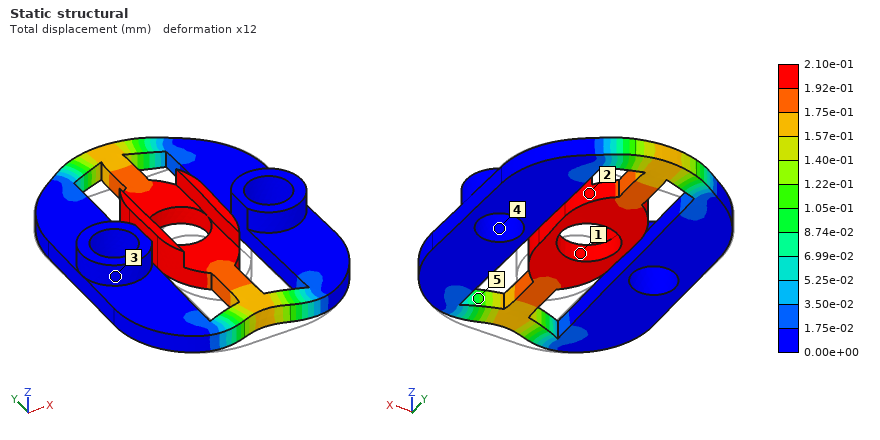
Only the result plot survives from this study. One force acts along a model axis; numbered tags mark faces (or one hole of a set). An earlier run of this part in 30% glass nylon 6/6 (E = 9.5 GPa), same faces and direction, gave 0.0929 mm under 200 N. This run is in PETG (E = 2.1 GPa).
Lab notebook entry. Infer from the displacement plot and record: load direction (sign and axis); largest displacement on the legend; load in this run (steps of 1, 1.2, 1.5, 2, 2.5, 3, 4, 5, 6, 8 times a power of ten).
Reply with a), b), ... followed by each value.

a) +Y
b) 2.10e-01 mm
c) 100 N
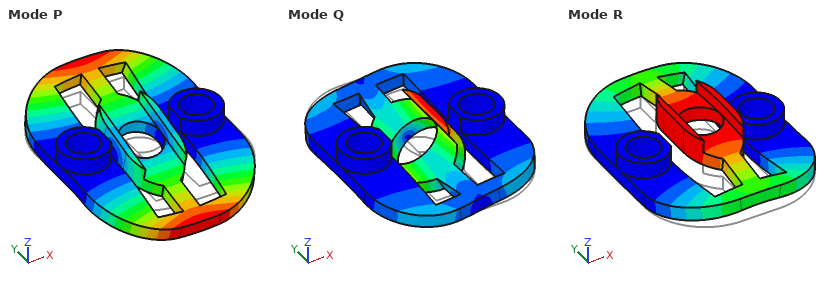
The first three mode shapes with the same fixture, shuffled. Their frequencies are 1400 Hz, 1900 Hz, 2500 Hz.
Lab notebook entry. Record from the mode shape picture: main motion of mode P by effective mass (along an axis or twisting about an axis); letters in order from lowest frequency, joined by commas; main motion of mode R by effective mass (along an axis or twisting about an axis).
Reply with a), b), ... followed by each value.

a) twisting about X
b) R, P, Q
c) along Z
